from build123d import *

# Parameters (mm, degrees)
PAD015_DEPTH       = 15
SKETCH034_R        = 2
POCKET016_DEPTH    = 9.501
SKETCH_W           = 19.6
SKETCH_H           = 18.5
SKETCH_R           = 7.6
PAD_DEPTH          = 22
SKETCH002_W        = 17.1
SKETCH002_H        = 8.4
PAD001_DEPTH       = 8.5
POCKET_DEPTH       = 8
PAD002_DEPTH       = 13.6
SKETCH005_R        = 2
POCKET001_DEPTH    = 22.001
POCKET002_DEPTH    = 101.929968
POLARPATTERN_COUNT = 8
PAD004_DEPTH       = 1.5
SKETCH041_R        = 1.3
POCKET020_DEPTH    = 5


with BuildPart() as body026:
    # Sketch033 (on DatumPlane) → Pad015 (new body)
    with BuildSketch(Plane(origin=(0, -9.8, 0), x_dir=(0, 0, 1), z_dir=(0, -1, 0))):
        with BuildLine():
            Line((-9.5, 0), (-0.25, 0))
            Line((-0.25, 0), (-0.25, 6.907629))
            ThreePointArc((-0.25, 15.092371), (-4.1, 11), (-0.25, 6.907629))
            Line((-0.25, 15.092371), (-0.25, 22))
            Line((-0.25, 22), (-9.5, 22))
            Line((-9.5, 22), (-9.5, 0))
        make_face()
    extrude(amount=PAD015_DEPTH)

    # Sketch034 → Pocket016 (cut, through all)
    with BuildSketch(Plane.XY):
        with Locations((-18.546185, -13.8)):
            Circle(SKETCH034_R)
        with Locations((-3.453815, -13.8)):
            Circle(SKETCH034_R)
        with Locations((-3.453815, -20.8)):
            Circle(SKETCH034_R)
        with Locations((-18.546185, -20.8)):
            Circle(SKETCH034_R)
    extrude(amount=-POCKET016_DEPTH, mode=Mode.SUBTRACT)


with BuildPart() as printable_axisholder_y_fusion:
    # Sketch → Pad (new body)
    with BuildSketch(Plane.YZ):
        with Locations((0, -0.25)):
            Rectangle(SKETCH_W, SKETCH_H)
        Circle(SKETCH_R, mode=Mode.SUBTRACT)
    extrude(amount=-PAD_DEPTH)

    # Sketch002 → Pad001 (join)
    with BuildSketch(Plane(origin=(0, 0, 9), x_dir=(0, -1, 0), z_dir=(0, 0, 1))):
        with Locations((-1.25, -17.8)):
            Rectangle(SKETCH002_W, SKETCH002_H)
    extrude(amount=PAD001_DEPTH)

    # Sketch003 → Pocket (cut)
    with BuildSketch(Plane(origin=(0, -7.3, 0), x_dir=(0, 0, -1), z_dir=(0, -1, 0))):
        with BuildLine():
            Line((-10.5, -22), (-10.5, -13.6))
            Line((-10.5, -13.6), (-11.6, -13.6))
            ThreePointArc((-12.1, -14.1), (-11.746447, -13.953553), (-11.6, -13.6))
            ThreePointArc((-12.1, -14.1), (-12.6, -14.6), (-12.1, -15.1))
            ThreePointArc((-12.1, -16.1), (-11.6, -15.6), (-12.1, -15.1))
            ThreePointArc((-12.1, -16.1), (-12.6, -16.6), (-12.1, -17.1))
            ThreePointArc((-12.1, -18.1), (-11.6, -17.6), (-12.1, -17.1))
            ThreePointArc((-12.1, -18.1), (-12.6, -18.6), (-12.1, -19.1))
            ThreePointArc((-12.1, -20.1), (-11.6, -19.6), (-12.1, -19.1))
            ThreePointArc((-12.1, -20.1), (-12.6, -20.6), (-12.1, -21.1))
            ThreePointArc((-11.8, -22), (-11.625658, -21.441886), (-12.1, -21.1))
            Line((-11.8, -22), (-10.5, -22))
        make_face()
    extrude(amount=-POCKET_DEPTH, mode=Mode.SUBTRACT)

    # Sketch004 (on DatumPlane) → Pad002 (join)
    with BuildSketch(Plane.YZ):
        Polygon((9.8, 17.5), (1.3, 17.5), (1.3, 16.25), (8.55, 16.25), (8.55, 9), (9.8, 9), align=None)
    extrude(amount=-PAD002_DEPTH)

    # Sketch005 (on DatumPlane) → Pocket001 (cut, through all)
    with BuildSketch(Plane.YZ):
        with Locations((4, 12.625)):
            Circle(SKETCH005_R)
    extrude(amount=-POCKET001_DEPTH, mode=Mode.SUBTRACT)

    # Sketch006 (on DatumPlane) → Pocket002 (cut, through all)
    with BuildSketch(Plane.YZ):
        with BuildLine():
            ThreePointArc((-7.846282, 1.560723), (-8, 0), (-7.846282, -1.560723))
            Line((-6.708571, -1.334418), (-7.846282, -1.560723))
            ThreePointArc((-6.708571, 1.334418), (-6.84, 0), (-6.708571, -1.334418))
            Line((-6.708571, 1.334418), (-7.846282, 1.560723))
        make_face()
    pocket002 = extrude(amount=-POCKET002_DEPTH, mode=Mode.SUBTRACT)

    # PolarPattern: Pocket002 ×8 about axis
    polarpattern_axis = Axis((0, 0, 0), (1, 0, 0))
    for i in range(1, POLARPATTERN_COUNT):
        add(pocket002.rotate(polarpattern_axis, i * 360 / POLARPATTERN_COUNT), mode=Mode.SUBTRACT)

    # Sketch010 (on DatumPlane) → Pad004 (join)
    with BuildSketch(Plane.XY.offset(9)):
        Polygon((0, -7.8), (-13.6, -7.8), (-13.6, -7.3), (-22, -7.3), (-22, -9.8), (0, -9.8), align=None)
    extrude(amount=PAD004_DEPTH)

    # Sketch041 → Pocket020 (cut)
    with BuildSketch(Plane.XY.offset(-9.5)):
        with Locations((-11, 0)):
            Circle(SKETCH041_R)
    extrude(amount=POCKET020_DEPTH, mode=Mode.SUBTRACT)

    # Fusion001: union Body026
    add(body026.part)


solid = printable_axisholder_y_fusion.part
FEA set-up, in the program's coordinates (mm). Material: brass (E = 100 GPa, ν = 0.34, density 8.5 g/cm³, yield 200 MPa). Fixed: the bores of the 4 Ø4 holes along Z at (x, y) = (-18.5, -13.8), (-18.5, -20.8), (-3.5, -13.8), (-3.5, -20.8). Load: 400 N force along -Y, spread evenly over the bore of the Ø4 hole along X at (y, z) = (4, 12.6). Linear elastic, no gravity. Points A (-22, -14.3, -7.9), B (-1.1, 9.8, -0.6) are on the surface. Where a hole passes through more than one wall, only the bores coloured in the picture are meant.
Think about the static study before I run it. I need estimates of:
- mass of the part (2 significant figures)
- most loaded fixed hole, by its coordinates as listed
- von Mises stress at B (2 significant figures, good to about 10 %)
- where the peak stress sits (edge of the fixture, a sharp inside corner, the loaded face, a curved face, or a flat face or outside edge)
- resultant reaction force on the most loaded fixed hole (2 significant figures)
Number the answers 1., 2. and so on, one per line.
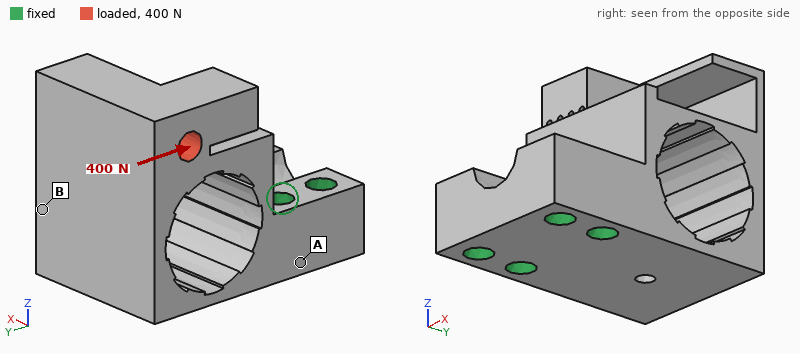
1. 62 g
2. (-18.5, -13.8)
3. 49 MPa
4. a curved face
5. 390 N
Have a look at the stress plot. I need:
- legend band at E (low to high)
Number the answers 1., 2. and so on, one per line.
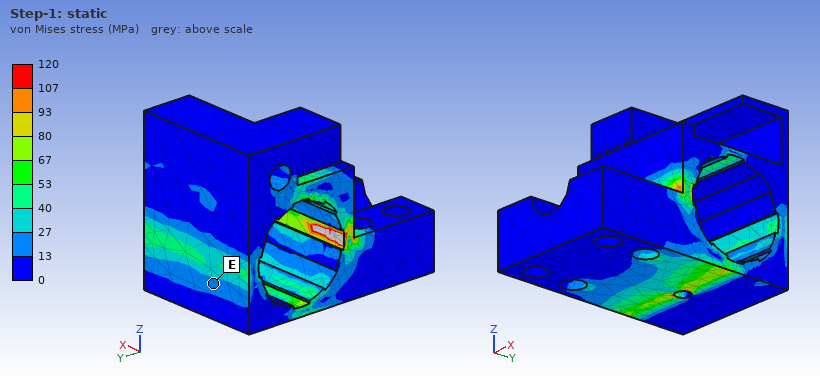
1. 13 to 27 MPa
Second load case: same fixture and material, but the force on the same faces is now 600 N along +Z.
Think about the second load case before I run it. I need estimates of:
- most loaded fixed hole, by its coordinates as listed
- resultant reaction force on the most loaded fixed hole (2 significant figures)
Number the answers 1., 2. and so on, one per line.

1. (-18.5, -13.8)
2. 580 N
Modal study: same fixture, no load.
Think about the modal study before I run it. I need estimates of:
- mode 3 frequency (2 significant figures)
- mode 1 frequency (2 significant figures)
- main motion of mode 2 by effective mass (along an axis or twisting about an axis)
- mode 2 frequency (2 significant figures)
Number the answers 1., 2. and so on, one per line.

1. 7800 Hz
2. 2100 Hz
3. along X
4. 4600 Hz
